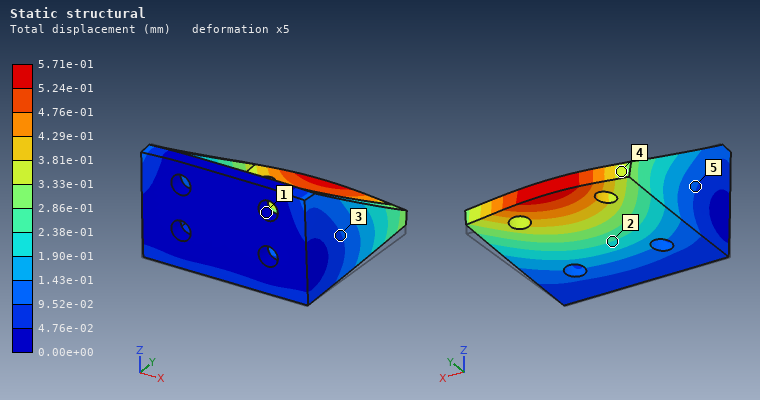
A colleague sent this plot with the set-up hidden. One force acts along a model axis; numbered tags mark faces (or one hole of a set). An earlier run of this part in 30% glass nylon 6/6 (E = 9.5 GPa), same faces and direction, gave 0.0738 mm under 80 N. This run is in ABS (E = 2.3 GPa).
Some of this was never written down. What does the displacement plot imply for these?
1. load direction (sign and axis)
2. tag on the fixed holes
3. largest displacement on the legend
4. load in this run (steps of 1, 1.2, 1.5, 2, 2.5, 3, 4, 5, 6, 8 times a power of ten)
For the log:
+Z
1
5.71e-01 mm
150 N
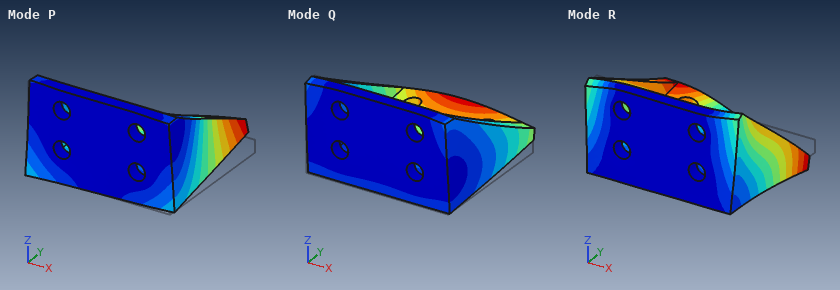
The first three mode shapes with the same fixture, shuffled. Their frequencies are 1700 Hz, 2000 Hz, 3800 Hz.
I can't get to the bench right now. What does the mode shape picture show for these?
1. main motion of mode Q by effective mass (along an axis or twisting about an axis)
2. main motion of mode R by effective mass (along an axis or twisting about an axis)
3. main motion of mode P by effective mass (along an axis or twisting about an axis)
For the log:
along Z
along X
along X
